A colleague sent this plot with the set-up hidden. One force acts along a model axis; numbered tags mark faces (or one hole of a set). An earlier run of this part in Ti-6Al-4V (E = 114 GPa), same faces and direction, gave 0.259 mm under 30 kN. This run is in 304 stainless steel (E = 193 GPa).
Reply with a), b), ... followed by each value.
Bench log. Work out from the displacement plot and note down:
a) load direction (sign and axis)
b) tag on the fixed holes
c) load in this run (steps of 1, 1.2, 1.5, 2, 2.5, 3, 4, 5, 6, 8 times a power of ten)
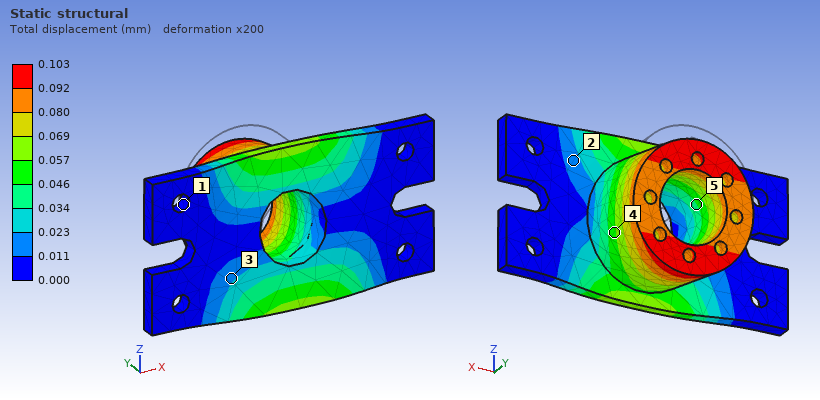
a) -Z
b) 1
c) 20 kN
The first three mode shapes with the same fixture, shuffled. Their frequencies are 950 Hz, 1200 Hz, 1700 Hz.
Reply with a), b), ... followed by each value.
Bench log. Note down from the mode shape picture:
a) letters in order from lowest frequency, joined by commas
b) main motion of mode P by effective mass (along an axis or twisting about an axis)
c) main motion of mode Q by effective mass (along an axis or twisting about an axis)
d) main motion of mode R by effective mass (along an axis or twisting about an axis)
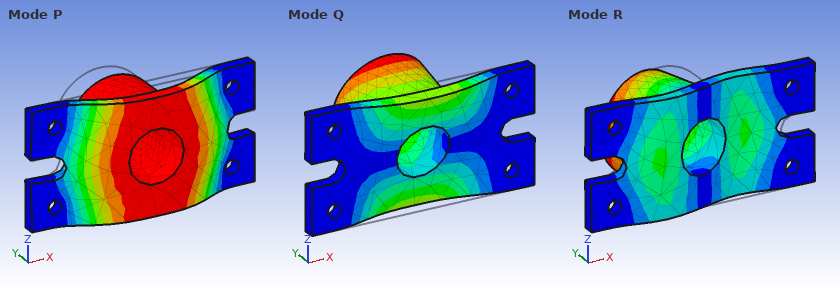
a) Q, P, R
b) along Y
c) along Z
d) along X
